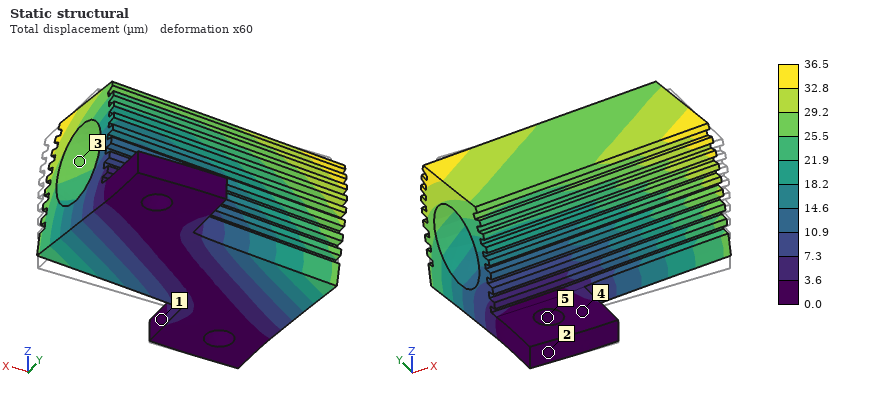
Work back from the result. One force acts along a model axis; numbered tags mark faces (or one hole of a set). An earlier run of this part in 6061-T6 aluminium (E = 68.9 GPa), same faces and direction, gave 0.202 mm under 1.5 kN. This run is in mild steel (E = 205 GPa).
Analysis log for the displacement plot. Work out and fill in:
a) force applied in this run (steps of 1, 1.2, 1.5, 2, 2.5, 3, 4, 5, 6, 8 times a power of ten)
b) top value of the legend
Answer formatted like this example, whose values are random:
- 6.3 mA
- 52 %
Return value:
- 800 N
- 36.5 µm
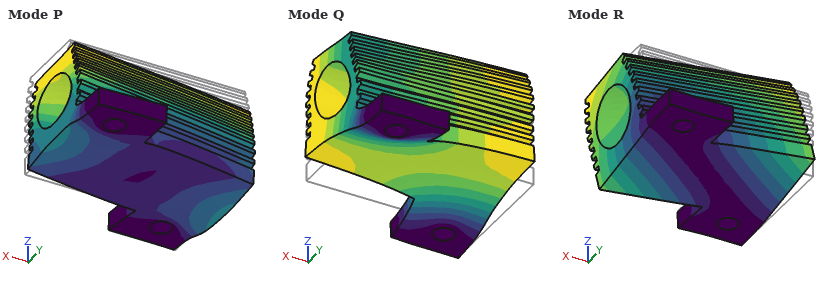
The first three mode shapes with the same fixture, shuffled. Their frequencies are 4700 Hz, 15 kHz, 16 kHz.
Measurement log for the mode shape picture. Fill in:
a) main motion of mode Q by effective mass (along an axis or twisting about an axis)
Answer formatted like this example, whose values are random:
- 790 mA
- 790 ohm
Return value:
- along Z
